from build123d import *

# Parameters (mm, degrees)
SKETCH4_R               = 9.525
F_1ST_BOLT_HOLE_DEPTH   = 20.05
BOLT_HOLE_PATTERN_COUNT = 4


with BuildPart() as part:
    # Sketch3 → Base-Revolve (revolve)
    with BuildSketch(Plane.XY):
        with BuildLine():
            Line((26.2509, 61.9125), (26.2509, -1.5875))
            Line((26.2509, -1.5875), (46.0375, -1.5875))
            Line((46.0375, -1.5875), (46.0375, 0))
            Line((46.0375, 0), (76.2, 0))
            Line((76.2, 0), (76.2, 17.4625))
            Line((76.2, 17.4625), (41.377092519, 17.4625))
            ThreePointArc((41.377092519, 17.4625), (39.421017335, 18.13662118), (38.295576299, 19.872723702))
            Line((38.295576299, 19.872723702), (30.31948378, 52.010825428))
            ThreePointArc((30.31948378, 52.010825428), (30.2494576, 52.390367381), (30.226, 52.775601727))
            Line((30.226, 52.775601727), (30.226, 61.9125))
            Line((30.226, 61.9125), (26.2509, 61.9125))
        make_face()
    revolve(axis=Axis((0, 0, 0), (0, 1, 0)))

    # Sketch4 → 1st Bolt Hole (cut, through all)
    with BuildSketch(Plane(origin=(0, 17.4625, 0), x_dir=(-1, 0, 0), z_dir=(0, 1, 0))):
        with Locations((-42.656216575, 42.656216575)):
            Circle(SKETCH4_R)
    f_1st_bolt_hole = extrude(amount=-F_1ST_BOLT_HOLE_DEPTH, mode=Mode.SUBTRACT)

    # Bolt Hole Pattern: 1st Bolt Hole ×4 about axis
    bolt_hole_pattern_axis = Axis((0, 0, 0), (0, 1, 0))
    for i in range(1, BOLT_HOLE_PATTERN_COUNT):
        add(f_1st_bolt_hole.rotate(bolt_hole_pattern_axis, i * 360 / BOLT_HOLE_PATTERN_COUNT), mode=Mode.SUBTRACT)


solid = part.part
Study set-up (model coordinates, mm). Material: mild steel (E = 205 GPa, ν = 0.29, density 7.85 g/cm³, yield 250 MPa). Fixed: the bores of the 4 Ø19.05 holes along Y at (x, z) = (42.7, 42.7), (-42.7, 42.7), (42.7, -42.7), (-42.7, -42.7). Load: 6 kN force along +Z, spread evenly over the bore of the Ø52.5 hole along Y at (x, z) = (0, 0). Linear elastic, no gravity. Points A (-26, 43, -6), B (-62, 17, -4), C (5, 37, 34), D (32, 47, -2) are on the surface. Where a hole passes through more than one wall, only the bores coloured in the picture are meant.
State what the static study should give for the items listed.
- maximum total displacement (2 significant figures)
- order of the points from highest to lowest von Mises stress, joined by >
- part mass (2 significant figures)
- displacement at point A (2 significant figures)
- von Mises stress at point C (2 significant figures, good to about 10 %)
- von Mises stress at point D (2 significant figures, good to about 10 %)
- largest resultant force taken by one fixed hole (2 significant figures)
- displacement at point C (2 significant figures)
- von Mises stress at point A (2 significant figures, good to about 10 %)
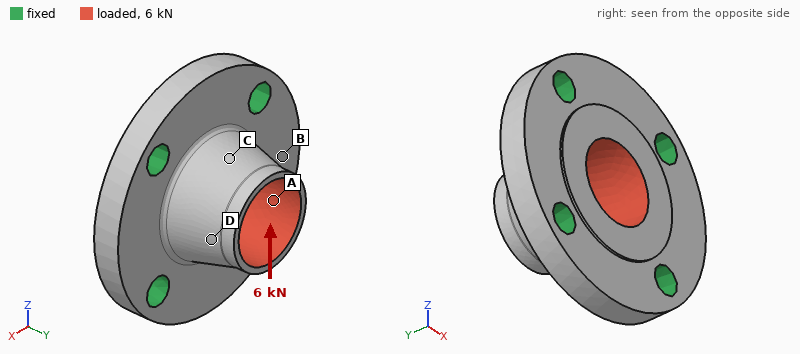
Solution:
3.3 µm
A > D > C > B
2.6 kg
1.7 µm
2.7 MPa
4.2 MPa
1.7 kN
1.8 µm
6.2 MPa
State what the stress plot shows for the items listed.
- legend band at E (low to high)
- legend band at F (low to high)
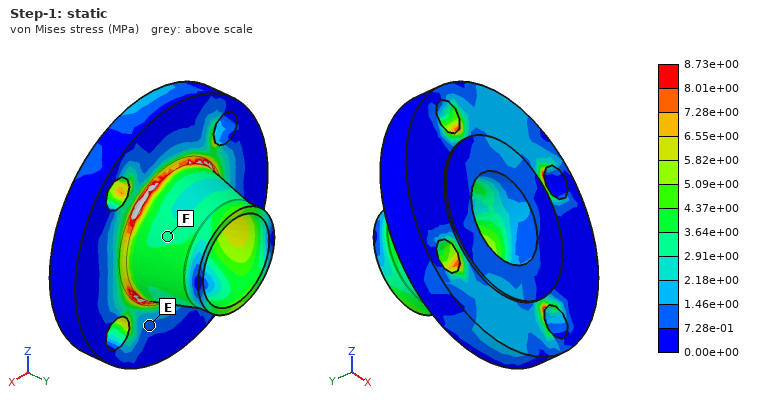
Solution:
7.28e-01 to 1.46e+00 MPa
2.91e+00 to 3.64e+00 MPa
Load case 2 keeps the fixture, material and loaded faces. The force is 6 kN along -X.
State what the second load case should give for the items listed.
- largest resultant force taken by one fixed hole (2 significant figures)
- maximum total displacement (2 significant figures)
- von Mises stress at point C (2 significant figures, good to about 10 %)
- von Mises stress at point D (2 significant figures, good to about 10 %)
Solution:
1.7 kN
3.3 µm
3.9 MPa
3.2 MPa
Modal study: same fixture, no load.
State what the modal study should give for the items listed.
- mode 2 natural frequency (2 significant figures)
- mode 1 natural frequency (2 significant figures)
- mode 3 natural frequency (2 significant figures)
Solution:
9800 Hz
8900 Hz
9800 Hz
